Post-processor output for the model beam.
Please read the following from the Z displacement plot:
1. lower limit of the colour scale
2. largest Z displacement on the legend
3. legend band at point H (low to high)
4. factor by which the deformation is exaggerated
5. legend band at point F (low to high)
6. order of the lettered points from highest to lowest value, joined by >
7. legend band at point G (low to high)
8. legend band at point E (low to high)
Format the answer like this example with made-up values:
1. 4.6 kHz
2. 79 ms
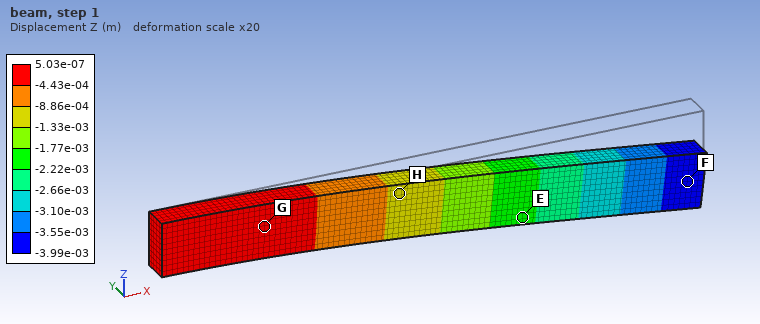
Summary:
1. -3.99e-03 m
2. 5.03e-07 m
3. -1.33e-03 to -8.86e-04 m
4. 20
5. -3.99e-03 to -3.55e-03 m
6. G > H > E > F
7. -4.43e-04 to 5.03e-07 m
8. -2.22e-03 to -1.77e-03 m
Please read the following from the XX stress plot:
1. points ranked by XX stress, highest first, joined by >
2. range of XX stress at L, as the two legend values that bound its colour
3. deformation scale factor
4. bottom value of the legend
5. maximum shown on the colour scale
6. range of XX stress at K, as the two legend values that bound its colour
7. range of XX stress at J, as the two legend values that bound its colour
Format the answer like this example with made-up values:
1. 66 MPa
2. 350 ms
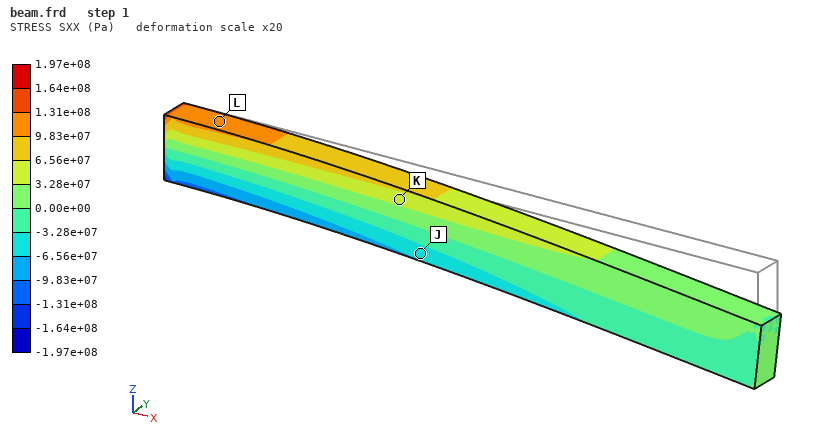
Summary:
1. L > K > J
2. 9.83e+07 to 1.31e+08 Pa
3. 20
4. -1.97e+08 Pa
5. 1.97e+08 Pa
6. 3.28e+07 to 6.56e+07 Pa
7. -6.56e+07 to -3.28e+07 Pa
